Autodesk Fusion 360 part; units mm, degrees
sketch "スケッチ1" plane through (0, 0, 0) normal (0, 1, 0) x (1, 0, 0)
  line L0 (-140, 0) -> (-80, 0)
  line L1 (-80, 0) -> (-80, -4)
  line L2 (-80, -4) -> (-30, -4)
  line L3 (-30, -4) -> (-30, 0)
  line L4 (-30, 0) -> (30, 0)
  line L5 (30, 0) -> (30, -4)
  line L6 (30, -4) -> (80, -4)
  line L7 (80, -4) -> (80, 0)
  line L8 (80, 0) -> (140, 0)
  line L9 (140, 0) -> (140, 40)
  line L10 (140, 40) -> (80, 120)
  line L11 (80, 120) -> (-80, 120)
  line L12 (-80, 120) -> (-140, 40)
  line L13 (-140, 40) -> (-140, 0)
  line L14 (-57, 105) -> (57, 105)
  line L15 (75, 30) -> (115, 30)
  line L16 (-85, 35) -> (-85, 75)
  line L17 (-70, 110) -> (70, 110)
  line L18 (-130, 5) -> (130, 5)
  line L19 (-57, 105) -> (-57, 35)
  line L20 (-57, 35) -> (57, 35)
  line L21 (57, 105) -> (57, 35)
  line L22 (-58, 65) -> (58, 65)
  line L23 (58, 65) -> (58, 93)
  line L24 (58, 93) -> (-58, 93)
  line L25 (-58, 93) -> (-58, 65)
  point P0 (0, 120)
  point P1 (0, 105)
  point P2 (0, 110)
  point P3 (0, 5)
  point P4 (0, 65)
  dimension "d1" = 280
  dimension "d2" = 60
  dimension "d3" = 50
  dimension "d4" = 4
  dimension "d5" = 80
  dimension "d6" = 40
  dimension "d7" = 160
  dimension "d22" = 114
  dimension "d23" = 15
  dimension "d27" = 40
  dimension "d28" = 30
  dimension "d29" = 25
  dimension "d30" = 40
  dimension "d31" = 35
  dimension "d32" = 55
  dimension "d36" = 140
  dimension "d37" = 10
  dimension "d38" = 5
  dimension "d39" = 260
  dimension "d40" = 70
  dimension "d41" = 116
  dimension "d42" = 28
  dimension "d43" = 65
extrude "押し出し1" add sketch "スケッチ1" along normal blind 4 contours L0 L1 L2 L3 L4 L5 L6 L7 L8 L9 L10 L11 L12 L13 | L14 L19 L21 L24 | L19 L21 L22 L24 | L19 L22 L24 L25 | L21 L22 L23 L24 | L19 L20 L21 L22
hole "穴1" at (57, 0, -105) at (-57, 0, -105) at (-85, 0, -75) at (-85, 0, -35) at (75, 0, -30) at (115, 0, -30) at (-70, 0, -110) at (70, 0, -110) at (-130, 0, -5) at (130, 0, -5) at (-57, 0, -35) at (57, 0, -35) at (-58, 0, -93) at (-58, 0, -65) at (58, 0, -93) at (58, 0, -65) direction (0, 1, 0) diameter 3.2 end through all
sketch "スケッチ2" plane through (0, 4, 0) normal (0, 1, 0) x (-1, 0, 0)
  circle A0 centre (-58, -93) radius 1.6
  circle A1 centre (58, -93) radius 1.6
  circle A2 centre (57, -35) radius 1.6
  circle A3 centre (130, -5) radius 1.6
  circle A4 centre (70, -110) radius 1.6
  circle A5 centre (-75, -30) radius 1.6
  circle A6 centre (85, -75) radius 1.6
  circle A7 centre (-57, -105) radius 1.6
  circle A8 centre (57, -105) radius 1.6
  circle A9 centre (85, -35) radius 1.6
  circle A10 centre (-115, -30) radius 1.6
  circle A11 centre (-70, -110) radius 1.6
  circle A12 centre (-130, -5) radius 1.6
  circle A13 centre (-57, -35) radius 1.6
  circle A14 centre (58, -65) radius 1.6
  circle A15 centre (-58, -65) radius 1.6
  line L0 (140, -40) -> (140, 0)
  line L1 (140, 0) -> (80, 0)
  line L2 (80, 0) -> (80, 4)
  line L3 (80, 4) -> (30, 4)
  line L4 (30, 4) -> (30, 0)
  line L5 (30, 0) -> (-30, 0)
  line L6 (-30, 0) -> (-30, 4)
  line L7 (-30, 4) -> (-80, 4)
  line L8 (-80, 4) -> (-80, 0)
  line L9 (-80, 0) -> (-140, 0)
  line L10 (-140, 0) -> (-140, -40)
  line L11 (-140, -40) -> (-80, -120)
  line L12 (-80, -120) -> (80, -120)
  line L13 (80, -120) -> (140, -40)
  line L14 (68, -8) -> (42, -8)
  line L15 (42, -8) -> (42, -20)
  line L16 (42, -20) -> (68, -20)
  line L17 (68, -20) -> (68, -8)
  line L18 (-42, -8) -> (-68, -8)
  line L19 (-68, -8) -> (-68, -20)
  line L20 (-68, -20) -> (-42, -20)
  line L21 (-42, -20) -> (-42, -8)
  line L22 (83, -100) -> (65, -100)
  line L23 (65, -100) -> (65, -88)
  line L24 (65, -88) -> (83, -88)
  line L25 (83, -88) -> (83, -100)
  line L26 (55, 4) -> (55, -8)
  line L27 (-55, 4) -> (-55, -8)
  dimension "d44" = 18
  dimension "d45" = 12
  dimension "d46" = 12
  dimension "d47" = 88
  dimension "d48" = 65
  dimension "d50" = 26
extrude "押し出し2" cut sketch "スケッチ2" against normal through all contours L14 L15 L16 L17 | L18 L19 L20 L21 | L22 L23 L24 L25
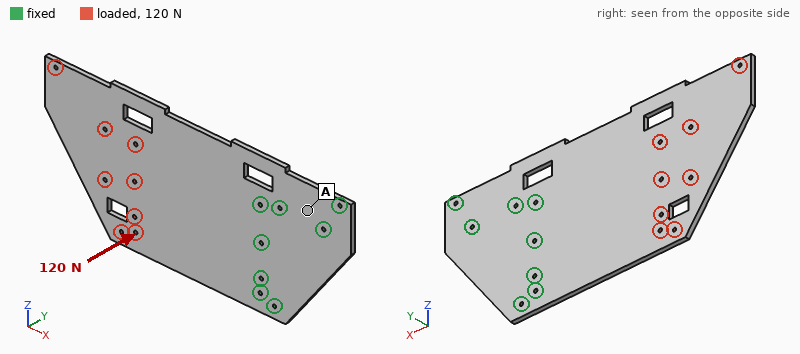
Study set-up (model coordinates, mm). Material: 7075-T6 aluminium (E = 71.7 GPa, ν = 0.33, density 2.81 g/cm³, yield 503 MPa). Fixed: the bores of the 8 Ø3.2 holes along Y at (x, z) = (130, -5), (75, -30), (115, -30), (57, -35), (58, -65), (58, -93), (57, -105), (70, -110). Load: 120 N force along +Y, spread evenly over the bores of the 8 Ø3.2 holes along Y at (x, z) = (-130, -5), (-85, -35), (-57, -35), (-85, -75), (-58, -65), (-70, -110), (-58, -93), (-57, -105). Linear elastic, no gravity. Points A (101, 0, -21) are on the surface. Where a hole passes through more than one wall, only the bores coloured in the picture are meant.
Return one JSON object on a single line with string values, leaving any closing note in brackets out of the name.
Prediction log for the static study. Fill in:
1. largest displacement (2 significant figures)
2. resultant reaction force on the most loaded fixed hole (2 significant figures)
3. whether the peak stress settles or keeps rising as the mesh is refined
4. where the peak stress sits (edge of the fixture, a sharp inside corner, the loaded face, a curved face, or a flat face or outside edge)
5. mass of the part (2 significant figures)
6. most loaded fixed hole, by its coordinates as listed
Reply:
{"largest displacement": "3.6 mm", "resultant reaction force on the most loaded fixed hole": "220 N", "whether the peak stress settles or keeps rising as the mesh is refined": "keeps rising", "where the peak stress sits": "edge of the fixture", "mass of the part": "320 g", "most loaded fixed hole, by its coordinates as listed": "(57, -35)"}
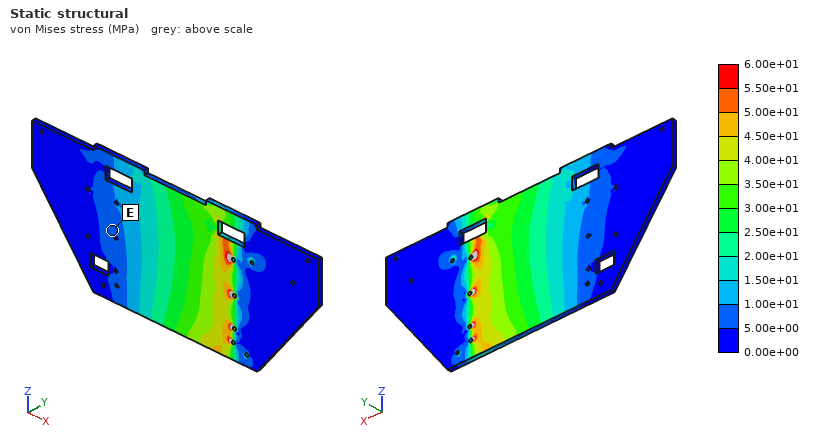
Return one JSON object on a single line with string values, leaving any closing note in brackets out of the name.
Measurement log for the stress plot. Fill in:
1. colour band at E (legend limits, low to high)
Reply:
{"colour band at E": "5.00e+00 to 1.00e+01 MPa"}
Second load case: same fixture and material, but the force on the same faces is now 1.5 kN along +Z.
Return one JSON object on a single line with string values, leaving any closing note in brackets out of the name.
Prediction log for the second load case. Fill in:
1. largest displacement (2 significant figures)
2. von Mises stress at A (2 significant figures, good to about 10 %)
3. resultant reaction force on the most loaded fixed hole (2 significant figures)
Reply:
{"largest displacement": "96 µm", "von Mises stress at A": "5.0 MPa", "resultant reaction force on the most loaded fixed hole": "1.4 kN"}
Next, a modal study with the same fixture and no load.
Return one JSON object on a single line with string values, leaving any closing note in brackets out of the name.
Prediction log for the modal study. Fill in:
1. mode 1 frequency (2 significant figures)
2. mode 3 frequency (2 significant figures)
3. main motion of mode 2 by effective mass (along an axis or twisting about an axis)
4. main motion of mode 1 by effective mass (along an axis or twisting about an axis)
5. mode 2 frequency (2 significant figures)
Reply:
{"mode 1 frequency": "100 Hz", "mode 3 frequency": "560 Hz", "main motion of mode 2 by effective mass": "twisting about X", "main motion of mode 1 by effective mass": "along Y", "mode 2 frequency": "360 Hz"}
